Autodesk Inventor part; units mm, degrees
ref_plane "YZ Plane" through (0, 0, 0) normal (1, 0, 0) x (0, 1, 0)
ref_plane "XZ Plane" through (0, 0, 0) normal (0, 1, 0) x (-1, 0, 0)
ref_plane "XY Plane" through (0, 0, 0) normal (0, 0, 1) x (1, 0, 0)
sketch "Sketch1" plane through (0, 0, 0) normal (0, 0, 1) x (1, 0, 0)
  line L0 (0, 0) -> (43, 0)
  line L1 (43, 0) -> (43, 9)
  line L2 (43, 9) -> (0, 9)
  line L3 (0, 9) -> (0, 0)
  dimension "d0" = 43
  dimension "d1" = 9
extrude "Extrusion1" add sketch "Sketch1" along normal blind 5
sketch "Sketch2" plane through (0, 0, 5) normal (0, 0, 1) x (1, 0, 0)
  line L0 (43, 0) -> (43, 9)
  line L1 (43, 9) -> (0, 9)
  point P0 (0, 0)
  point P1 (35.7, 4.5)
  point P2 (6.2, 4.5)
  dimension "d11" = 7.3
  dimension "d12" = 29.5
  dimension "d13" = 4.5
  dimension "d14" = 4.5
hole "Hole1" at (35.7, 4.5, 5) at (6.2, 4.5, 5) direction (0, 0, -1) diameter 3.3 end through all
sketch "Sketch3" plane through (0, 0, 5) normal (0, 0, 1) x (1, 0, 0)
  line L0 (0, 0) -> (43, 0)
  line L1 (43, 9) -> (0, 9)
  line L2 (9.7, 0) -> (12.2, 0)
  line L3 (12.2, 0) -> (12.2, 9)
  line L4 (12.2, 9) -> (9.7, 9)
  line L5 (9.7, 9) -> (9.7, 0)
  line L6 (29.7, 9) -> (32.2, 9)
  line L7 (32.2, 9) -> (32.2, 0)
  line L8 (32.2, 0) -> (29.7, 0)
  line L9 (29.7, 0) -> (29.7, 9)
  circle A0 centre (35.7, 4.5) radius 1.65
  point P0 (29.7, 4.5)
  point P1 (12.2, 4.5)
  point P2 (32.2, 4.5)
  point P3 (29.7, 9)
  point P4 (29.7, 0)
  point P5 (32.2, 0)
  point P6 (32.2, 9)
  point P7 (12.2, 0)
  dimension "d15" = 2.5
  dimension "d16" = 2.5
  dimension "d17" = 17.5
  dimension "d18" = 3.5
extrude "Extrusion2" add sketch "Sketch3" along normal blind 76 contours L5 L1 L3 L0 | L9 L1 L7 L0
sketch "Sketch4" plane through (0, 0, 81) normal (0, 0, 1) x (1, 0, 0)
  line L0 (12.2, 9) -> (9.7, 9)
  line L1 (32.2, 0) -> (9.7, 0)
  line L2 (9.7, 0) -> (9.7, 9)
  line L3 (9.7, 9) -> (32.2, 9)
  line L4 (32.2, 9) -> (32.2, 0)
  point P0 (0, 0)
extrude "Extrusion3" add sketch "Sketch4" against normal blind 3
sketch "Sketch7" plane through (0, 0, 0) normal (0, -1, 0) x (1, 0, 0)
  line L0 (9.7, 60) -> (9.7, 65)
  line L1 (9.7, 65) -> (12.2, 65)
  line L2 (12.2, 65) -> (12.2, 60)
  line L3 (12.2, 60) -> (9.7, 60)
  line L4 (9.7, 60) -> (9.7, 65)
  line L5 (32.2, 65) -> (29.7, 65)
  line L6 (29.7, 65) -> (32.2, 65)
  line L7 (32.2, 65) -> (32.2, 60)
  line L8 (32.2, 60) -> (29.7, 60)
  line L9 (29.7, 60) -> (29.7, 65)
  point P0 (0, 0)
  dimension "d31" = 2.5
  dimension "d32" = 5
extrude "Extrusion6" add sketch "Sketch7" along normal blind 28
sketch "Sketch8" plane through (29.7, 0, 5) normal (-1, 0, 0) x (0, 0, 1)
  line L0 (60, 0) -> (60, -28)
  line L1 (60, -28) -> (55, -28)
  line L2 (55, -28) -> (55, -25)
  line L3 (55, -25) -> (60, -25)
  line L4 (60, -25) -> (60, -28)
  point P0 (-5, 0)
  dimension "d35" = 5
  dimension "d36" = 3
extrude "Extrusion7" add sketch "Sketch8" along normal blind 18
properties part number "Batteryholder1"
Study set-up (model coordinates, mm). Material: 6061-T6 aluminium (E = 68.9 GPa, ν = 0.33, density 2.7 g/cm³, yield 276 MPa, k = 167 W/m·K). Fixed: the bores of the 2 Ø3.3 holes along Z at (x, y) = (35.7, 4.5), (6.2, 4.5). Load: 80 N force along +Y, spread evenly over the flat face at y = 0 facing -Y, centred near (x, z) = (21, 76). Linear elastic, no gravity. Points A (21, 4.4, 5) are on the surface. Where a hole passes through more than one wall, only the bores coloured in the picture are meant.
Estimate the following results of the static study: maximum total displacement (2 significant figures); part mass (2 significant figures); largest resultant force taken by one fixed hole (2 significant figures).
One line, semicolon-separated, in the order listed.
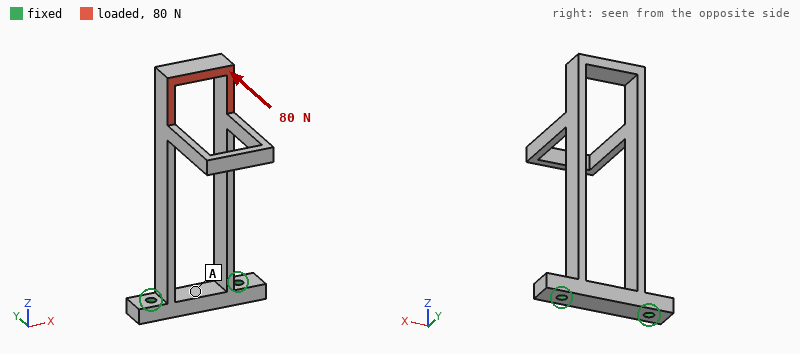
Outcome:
0.65 mm; 18 g; 40 N
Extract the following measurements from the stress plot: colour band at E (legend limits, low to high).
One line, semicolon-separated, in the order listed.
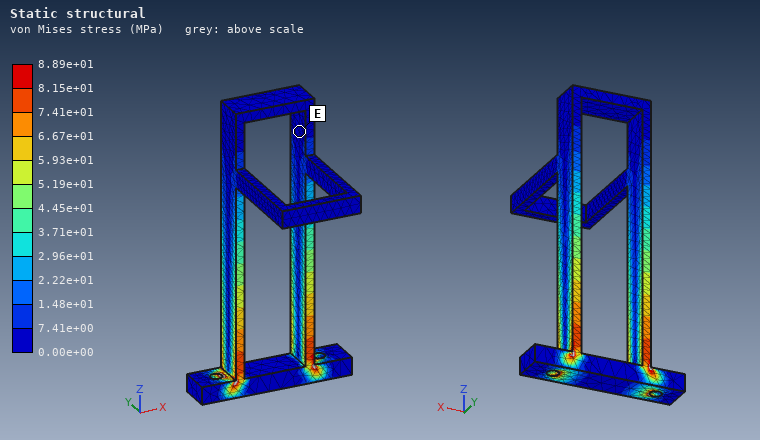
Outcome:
0.00e+00 to 7.41e+00 MPa
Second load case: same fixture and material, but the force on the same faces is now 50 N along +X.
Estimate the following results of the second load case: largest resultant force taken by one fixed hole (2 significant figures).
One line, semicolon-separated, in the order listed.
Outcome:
130 N
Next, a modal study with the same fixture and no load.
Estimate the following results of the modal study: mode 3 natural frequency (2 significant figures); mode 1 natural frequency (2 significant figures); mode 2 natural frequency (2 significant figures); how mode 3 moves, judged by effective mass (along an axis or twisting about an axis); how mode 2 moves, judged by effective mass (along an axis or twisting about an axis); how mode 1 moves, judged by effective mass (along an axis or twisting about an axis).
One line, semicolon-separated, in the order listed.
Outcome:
1000 Hz; 410 Hz; 730 Hz; twisting about Z; along Y; along X
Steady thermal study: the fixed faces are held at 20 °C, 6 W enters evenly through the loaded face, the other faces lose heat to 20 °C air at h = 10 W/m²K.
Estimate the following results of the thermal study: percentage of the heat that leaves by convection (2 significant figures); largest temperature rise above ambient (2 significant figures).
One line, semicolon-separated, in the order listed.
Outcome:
24 %; 49 K
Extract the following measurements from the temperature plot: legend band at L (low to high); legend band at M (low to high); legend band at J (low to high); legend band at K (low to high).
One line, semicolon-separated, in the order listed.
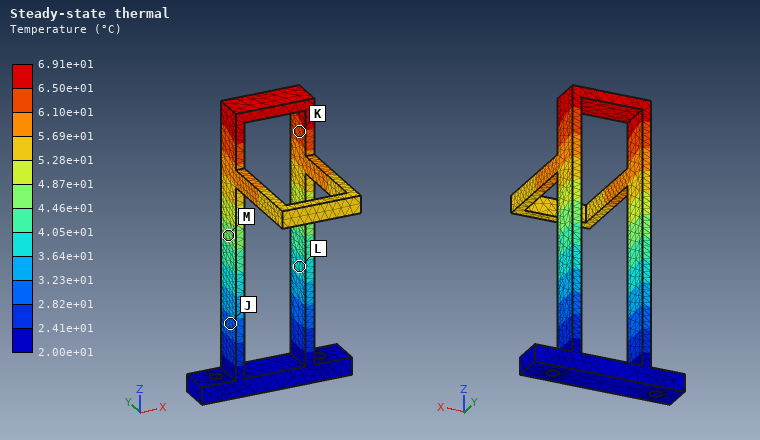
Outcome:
3.64e+01 to 4.05e+01 °C; 4.46e+01 to 4.87e+01 °C; 2.82e+01 to 3.23e+01 °C; 6.10e+01 to 6.50e+01 °C
